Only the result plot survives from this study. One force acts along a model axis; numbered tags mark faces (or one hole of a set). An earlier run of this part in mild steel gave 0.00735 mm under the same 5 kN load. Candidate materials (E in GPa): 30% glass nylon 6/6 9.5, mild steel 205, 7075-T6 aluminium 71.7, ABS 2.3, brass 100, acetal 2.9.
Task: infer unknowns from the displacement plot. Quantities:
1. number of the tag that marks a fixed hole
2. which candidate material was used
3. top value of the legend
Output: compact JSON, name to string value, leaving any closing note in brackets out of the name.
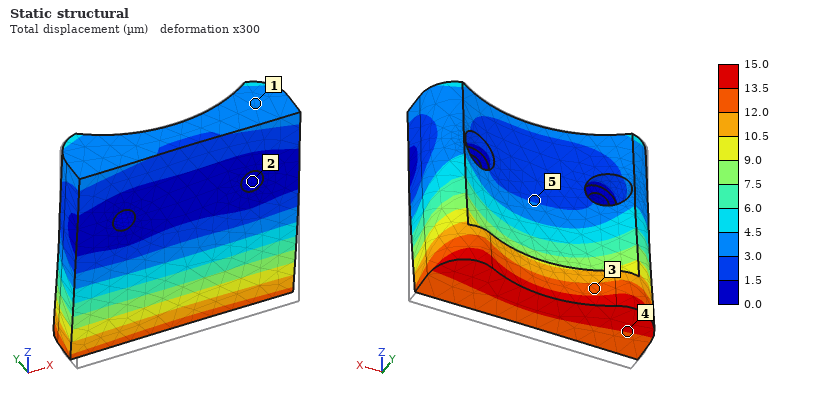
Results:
{"number of the tag that marks a fixed hole": "2", "which candidate material was used": "brass", "top value of the legend": "15.0 µm"}
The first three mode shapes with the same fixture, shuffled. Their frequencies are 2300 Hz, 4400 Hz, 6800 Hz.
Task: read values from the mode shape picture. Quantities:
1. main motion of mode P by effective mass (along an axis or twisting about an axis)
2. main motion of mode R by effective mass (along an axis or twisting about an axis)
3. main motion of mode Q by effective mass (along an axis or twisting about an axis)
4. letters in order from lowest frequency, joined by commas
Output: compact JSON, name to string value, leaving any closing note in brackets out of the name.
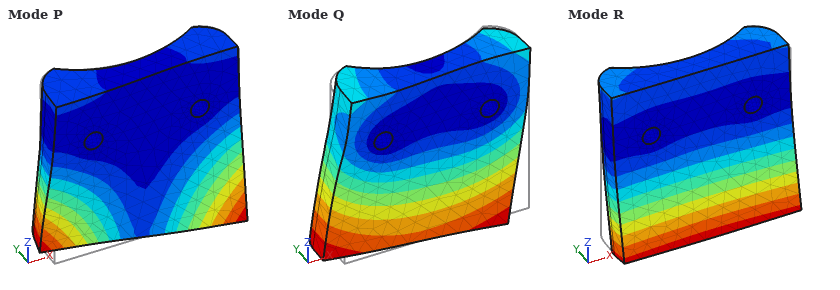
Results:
{"main motion of mode P by effective mass": "twisting about Z", "main motion of mode R by effective mass": "along Y", "main motion of mode Q by effective mass": "along X", "letters in order from lowest frequency, joined by commas": "R, P, Q"}
